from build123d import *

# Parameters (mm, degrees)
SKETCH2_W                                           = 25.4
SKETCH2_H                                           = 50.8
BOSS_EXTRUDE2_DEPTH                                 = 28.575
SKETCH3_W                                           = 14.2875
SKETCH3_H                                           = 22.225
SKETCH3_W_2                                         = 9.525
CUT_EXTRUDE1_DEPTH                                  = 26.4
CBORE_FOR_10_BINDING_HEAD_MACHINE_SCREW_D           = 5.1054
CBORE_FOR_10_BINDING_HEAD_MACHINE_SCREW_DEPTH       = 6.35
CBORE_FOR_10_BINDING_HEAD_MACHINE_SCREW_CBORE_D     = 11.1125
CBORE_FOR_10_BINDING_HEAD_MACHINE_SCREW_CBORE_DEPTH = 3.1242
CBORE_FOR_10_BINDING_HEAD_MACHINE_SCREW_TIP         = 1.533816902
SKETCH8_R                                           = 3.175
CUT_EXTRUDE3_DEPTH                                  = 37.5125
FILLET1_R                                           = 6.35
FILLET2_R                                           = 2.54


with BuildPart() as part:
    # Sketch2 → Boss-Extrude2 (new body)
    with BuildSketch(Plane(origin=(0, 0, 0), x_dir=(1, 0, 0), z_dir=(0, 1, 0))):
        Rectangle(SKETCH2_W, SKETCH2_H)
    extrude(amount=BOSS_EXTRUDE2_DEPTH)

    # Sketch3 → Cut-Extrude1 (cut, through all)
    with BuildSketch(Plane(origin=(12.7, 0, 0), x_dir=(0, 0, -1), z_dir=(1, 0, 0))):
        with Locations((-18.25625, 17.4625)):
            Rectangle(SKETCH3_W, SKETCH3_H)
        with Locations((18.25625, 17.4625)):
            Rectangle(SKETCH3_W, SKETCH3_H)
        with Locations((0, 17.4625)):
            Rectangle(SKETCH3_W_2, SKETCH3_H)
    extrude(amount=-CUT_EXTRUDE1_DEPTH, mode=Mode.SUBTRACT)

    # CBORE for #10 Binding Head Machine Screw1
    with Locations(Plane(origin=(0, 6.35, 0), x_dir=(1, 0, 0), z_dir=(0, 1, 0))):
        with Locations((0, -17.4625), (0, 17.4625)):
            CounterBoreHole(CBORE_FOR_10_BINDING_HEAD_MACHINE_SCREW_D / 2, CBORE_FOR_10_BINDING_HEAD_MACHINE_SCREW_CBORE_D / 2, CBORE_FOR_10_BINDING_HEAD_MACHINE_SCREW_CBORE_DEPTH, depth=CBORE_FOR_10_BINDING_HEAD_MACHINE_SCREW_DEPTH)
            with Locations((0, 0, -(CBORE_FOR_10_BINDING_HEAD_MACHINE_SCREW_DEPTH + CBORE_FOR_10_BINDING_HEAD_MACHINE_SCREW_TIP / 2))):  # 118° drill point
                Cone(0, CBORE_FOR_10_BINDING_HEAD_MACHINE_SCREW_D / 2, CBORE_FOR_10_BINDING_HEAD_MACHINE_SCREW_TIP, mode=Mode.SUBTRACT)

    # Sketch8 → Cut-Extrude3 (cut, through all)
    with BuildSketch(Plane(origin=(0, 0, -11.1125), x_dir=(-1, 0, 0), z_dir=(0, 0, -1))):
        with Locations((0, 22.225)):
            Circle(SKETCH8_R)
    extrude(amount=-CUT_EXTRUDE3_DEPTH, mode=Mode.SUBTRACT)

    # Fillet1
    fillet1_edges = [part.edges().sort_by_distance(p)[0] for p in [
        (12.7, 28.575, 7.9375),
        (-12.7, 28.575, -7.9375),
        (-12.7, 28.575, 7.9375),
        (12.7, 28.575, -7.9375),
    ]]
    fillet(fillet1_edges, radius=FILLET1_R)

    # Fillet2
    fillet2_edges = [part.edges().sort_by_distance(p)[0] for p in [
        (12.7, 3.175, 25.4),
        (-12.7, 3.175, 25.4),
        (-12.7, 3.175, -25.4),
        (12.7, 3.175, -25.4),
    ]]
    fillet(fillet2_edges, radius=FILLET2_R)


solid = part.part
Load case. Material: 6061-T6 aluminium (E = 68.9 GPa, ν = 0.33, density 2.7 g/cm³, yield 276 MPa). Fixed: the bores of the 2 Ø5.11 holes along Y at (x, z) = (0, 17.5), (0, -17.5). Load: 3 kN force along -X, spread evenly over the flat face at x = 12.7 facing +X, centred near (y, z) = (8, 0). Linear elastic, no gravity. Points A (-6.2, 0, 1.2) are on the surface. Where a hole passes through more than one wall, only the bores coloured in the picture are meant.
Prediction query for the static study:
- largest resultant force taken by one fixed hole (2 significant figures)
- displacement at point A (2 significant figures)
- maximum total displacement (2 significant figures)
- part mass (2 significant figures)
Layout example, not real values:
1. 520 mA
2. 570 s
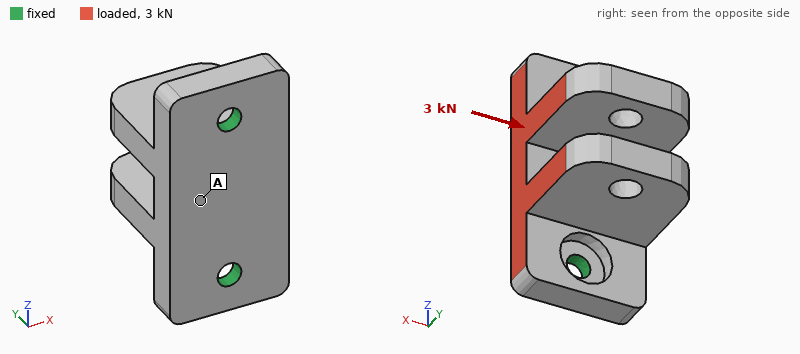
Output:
1. 1.5 kN
2. 0.022 mm
3. 0.11 mm
4. 38 g
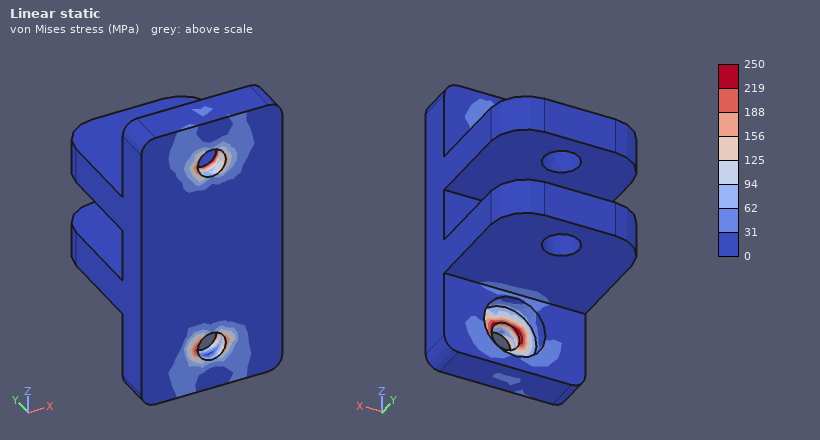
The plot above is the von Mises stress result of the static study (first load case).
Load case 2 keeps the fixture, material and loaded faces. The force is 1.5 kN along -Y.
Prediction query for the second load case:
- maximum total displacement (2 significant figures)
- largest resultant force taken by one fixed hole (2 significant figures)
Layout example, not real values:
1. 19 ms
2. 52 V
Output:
1. 0.10 mm
2. 850 N
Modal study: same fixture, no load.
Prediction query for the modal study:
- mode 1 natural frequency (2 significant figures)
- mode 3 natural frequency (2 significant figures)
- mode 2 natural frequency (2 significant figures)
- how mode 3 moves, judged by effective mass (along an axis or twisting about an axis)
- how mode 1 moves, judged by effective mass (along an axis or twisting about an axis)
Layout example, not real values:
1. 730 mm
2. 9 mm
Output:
1. 4300 Hz
2. 8500 Hz
3. 6600 Hz
4. along Z
5. along X
